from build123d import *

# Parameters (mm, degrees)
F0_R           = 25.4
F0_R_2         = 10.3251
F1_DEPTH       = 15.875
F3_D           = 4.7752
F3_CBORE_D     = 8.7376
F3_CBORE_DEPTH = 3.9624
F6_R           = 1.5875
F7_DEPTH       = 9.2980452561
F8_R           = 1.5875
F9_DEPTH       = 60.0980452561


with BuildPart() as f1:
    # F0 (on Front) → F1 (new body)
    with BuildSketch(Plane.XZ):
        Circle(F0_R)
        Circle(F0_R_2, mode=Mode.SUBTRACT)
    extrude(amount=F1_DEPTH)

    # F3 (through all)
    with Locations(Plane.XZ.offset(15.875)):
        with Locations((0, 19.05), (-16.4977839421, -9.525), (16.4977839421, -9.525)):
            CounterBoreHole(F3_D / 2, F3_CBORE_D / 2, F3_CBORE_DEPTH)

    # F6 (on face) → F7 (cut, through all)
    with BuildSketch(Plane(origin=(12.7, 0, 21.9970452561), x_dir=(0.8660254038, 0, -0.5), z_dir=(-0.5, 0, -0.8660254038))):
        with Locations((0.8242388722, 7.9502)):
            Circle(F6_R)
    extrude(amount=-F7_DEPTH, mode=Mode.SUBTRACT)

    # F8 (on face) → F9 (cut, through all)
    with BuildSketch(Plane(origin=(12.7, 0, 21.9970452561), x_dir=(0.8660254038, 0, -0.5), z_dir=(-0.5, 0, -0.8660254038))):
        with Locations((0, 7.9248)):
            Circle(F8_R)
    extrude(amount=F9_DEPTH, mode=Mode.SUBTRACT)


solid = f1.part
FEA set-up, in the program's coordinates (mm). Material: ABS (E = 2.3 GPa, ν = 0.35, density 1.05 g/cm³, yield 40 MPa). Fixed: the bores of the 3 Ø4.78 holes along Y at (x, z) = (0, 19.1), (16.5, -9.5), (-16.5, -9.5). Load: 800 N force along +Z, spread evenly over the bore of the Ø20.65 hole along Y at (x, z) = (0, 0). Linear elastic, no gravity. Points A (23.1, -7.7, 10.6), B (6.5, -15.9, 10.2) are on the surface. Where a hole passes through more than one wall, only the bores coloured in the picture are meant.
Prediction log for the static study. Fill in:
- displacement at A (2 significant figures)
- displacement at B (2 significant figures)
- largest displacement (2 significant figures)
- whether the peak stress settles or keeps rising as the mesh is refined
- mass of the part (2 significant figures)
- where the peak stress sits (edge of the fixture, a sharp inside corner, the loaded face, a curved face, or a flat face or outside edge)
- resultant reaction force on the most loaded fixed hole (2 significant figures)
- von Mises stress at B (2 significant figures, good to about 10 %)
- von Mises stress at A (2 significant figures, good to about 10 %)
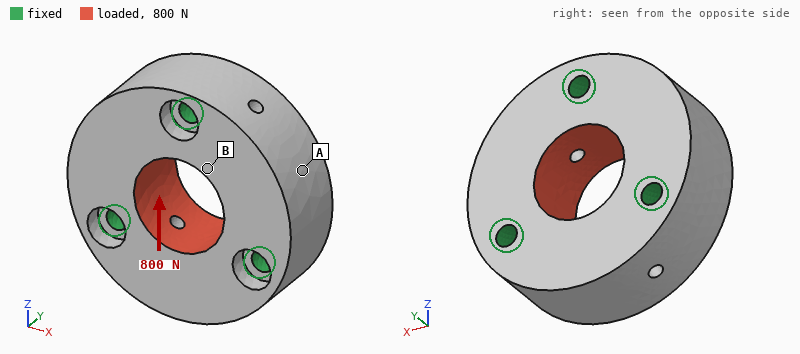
5.7 µm
9.0 µm
17 µm
keeps rising
27 g
edge of the fixture
290 N
1.2 MPa
0.43 MPa
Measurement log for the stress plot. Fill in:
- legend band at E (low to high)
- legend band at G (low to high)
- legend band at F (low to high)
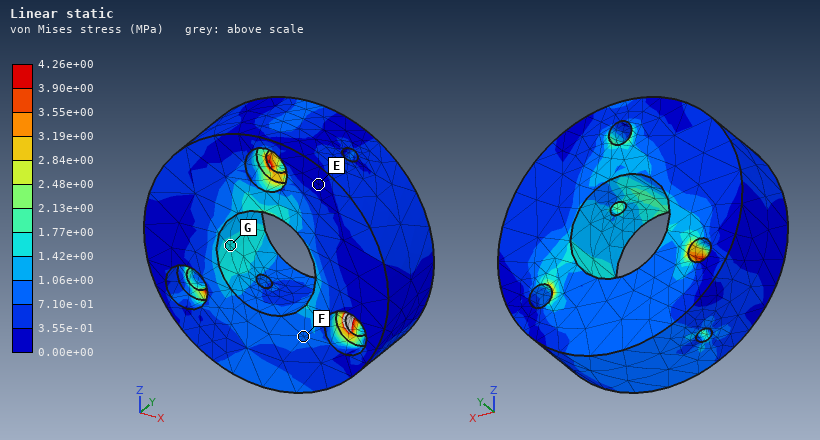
0.00e+00 to 3.55e-01 MPa
1.42e+00 to 1.77e+00 MPa
7.10e-01 to 1.06e+00 MPa
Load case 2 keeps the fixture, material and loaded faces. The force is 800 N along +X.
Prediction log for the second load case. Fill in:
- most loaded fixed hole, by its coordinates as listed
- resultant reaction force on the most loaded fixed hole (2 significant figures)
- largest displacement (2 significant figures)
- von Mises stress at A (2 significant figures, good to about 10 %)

(0, 19.1)
300 N
15 µm
0.75 MPa
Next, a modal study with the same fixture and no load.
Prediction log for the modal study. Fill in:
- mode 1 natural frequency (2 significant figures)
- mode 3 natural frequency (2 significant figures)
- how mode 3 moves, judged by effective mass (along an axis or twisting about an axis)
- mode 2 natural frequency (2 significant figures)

6300 Hz
7700 Hz
along Y
6400 Hz
